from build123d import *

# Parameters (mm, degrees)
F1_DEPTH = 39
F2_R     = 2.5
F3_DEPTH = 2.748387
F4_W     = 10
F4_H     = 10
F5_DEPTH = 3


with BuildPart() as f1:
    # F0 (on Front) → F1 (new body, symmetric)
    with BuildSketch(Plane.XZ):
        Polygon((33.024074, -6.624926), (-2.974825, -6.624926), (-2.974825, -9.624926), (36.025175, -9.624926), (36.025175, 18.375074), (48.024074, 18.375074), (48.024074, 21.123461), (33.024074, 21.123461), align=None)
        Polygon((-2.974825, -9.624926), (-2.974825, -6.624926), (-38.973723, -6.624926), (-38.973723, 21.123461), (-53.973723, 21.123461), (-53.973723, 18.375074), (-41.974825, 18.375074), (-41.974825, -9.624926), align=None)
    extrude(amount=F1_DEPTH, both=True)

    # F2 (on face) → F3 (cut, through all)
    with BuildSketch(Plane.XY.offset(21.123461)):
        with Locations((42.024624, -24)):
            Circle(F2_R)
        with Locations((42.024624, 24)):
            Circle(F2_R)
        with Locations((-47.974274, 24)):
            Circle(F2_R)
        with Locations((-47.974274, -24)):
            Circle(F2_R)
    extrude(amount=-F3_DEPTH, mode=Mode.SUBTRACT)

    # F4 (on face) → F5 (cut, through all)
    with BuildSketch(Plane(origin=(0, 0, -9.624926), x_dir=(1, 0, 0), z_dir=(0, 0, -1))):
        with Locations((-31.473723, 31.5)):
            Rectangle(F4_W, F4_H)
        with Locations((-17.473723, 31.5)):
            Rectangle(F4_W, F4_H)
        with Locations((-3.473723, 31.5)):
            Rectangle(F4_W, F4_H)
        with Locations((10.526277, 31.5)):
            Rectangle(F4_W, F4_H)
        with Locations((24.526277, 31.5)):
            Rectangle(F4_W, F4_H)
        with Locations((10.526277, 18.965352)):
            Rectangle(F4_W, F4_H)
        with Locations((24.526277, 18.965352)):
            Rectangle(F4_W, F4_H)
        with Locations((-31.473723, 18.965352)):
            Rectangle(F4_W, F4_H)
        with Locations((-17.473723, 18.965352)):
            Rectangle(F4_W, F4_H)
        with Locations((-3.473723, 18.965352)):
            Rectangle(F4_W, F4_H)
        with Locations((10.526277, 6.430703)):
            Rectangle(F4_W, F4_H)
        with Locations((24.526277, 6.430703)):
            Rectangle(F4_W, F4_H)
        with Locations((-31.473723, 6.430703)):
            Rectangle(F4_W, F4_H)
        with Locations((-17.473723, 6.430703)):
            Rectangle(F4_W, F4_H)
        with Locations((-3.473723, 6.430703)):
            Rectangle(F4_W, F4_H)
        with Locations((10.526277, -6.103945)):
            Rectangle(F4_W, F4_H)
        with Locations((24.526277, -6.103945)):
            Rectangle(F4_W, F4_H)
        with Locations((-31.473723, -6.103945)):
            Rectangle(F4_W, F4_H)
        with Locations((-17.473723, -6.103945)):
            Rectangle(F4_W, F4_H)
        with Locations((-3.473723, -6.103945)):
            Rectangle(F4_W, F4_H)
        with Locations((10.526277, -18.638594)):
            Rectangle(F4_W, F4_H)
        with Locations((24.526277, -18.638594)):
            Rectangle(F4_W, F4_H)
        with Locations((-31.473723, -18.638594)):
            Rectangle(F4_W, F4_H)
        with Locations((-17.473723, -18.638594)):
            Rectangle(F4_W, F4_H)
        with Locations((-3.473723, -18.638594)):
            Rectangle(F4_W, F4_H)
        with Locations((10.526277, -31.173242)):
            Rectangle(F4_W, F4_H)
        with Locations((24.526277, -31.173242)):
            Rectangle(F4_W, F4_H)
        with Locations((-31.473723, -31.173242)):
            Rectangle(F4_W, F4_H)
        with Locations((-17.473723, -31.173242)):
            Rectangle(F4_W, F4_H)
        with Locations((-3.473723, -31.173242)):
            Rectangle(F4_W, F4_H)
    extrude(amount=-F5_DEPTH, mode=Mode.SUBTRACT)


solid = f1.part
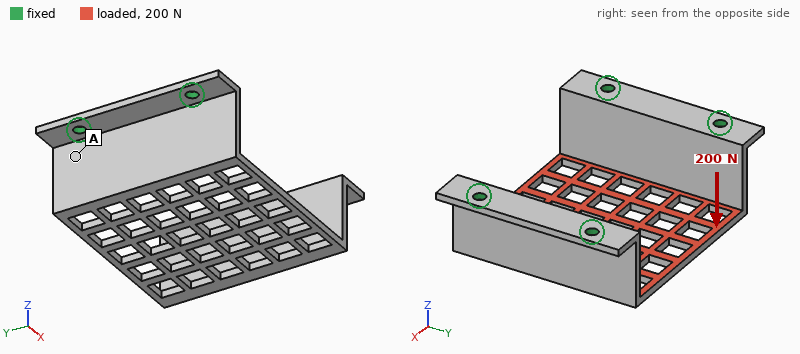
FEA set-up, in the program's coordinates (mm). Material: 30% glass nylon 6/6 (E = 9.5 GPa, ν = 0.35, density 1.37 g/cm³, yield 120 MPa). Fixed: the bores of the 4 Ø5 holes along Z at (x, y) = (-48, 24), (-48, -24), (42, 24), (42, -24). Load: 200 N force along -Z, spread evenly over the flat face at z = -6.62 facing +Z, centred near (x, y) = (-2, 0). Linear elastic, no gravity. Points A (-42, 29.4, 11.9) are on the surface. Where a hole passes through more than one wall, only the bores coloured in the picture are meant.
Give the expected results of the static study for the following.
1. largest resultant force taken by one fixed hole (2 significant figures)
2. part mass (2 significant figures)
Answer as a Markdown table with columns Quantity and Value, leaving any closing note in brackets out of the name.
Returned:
| Quantity | Value |
|---|---|
| largest resultant force taken by one fixed hole | 60 N |
| part mass | 37 g |
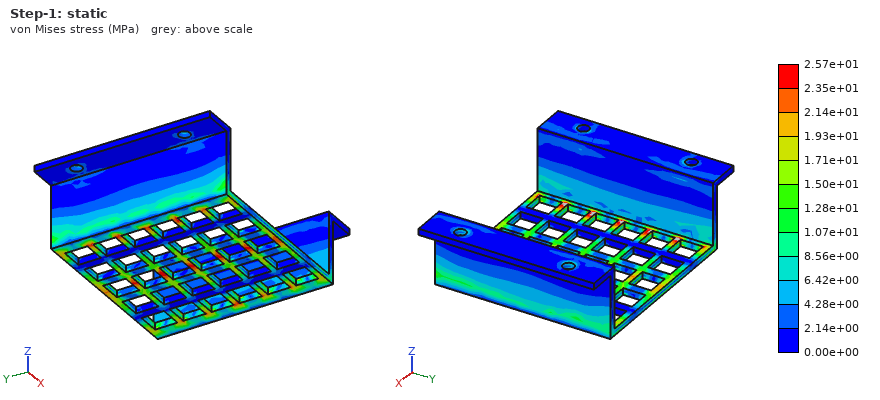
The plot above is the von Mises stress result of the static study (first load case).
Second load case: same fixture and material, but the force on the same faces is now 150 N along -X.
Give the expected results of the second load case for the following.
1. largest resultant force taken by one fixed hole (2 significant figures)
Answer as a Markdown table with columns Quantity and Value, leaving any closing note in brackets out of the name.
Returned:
| Quantity | Value |
|---|---|
| largest resultant force taken by one fixed hole | 39 N |
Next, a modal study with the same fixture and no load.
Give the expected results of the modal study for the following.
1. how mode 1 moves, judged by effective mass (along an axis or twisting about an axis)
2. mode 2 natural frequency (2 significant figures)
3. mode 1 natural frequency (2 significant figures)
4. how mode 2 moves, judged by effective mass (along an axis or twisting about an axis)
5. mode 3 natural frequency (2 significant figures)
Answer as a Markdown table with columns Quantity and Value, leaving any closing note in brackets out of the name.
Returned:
| Quantity | Value |
|---|---|
| how mode 1 moves, judged by effective mass | along X |
| mode 2 natural frequency | 1100 Hz |
| mode 1 natural frequency | 710 Hz |
| how mode 2 moves, judged by effective mass | along Z |
| mode 3 natural frequency | 1300 Hz |
